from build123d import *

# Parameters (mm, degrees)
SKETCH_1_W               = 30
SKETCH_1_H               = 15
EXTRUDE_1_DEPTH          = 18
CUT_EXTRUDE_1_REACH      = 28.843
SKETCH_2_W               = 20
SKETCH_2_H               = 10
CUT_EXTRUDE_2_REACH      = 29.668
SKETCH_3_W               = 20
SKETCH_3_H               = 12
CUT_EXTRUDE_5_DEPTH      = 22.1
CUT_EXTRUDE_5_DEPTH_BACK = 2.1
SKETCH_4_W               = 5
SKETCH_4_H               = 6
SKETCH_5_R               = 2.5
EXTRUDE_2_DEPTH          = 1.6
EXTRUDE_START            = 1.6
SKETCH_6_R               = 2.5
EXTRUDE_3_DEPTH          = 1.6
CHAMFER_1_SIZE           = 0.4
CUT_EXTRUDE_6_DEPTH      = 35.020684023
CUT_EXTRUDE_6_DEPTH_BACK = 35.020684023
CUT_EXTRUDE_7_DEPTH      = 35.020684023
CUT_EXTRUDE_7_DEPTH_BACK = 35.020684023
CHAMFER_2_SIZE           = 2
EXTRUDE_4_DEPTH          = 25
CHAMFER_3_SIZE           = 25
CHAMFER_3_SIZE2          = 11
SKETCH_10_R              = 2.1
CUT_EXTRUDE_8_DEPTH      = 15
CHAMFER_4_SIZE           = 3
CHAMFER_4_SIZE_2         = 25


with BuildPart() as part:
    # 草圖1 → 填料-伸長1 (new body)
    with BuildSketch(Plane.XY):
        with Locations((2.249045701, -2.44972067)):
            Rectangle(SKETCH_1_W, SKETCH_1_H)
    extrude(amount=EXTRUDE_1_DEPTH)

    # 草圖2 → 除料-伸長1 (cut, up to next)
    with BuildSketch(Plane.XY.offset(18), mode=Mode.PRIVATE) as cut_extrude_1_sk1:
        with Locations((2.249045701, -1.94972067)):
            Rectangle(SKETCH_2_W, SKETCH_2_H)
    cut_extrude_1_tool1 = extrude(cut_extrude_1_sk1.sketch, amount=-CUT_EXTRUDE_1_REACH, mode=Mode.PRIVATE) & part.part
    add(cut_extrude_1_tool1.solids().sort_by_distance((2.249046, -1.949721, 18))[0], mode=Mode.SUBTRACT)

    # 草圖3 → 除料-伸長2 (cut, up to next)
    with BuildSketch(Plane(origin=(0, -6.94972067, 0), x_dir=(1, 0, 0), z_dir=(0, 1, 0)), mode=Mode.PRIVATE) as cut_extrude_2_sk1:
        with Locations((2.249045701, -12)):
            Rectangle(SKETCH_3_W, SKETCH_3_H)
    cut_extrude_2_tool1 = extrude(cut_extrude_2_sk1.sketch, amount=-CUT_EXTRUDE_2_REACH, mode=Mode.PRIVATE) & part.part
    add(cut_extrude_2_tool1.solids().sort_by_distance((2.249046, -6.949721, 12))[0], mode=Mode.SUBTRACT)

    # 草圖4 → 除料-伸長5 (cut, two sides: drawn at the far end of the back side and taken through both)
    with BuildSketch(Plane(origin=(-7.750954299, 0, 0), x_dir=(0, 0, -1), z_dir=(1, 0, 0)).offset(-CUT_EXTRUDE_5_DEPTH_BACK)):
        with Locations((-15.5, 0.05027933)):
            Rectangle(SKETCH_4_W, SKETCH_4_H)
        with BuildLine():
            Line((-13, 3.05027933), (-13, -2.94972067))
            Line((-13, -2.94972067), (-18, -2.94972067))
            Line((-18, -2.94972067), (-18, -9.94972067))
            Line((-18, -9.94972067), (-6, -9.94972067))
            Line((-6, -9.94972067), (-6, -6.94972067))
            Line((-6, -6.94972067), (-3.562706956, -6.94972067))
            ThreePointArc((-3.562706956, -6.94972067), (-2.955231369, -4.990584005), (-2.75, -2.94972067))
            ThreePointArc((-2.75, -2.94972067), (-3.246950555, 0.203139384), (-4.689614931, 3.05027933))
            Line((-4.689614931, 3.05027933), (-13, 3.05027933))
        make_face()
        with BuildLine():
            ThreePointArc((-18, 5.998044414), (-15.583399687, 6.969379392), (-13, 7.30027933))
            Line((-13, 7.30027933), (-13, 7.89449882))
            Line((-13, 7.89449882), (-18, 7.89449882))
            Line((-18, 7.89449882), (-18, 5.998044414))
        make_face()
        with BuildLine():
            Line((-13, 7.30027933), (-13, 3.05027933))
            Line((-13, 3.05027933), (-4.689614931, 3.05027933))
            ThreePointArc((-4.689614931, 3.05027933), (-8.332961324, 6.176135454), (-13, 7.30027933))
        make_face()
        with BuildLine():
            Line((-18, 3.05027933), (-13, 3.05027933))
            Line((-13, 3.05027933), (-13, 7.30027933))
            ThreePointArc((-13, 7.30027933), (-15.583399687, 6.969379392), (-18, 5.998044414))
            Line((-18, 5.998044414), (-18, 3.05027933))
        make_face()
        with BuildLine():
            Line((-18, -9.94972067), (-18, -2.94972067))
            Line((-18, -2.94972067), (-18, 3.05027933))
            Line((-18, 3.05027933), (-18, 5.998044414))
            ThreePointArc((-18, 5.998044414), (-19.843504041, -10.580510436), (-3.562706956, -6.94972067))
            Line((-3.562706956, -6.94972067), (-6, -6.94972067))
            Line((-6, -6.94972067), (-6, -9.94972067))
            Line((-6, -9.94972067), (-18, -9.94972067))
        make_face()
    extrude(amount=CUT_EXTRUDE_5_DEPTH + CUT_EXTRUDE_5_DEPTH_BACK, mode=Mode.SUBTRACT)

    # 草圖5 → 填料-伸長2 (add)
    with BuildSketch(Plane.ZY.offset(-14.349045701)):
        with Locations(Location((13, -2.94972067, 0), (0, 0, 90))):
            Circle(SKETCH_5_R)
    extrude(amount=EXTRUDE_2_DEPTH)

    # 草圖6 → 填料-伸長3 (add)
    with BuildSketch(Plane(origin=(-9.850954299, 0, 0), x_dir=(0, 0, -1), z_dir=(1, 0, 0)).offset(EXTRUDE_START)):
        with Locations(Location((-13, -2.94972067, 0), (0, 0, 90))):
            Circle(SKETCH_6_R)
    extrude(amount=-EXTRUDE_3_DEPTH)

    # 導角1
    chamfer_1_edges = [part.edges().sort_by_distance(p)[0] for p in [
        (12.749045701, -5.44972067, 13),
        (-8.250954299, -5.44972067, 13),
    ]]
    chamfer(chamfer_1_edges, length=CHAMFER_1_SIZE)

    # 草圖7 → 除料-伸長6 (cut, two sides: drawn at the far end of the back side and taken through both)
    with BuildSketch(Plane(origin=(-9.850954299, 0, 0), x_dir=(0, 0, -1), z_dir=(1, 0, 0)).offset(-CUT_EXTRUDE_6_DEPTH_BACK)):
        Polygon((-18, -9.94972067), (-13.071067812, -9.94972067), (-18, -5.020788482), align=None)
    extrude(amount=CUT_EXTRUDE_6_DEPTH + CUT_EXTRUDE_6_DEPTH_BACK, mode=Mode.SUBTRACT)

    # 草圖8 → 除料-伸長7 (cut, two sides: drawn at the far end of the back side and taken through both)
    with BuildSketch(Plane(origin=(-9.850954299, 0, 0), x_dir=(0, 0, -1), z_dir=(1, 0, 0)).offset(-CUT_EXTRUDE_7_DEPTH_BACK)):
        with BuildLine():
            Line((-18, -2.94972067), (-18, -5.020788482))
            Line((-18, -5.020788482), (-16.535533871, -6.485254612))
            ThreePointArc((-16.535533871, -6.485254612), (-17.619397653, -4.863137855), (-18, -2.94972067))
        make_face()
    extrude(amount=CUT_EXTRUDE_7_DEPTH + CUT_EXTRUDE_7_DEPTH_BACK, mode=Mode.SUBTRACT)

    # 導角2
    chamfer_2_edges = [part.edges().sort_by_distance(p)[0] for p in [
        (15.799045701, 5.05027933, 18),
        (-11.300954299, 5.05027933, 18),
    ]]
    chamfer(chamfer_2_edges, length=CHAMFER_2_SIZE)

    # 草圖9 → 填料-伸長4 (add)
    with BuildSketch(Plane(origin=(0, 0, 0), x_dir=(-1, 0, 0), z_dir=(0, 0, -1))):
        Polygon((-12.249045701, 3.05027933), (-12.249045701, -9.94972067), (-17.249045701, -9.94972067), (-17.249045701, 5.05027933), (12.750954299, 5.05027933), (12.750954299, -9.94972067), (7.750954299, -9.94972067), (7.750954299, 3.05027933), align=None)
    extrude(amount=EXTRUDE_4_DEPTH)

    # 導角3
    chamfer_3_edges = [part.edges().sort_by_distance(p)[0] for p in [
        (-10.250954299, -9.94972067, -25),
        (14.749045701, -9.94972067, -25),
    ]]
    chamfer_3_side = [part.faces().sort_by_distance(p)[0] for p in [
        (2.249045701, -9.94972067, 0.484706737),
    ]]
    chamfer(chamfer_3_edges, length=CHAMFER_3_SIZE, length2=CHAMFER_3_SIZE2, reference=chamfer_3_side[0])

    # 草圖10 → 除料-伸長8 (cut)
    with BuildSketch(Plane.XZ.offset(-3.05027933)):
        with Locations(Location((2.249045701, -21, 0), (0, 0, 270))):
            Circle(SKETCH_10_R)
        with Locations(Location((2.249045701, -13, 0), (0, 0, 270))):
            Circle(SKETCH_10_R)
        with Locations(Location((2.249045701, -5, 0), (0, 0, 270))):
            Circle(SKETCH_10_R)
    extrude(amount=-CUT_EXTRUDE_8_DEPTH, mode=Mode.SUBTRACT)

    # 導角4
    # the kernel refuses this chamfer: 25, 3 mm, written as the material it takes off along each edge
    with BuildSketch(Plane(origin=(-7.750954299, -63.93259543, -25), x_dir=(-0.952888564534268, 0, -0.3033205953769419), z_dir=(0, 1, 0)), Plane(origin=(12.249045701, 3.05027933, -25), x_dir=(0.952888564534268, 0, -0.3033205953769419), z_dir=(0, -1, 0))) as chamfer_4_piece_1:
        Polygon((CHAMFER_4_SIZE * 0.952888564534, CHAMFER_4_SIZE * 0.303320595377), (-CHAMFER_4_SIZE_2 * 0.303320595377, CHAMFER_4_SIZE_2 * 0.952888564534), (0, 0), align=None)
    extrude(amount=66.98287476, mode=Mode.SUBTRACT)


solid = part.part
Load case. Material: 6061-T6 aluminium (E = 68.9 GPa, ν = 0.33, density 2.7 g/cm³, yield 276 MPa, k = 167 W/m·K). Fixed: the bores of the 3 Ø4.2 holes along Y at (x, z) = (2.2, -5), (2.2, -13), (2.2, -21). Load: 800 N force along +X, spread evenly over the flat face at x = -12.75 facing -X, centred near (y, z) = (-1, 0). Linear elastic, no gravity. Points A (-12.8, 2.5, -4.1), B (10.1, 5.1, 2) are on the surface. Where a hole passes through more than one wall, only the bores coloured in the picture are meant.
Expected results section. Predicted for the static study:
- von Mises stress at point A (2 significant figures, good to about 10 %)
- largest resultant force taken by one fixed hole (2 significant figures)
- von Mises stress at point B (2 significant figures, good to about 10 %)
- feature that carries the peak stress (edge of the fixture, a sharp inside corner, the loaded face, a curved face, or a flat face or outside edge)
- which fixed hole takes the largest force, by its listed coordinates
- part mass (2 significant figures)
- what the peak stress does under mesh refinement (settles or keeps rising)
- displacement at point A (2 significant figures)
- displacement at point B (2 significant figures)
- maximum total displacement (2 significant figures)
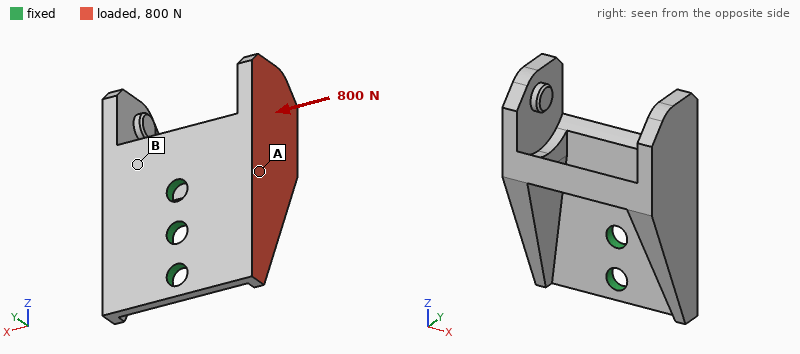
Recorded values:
21 MPa
860 N
63 MPa
edge of the fixture
(2.2, -5)
14 g
keeps rising
0.12 mm
0.043 mm
0.27 mm
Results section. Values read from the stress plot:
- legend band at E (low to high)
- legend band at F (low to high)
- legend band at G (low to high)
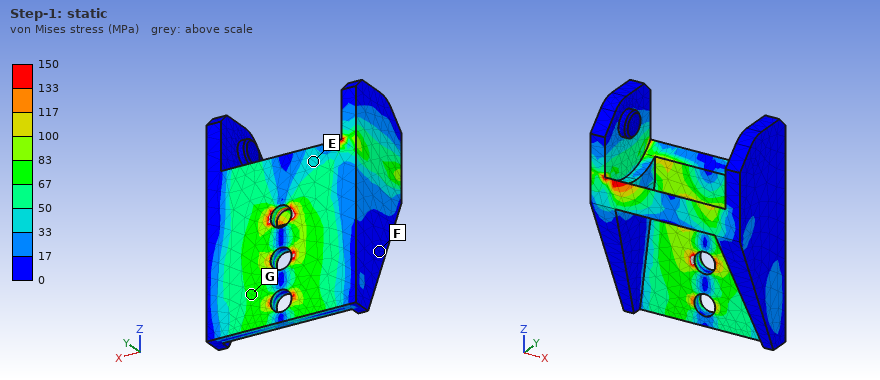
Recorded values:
33 to 50 MPa
0 to 17 MPa
67 to 83 MPa
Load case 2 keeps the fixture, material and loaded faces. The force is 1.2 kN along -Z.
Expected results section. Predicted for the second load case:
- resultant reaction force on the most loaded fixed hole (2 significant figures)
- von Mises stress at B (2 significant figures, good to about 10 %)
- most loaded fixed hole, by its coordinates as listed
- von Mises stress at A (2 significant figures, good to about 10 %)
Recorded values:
1.1 kN
34 MPa
(2.2, -5)
28 MPa
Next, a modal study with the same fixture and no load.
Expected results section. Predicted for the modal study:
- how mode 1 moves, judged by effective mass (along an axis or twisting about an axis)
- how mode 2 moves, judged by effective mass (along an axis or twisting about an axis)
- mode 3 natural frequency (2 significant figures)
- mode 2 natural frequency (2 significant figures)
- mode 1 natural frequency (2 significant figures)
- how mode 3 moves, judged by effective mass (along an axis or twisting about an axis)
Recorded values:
along X
along Y
5600 Hz
3600 Hz
2400 Hz
along X
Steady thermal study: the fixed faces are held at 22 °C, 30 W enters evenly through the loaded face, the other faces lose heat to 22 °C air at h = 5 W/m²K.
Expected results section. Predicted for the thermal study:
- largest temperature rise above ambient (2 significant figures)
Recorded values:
55 K
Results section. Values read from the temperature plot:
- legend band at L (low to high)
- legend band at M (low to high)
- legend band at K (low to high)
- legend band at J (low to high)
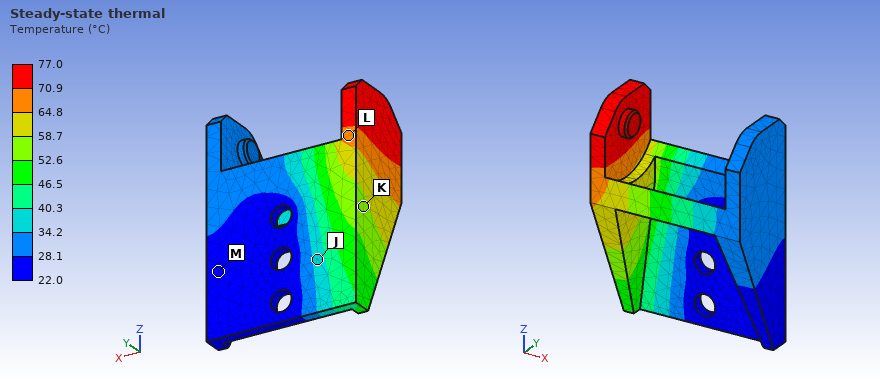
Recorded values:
64.8 to 70.9 °C
22.0 to 28.1 °C
52.6 to 58.7 °C
34.2 to 40.3 °C
